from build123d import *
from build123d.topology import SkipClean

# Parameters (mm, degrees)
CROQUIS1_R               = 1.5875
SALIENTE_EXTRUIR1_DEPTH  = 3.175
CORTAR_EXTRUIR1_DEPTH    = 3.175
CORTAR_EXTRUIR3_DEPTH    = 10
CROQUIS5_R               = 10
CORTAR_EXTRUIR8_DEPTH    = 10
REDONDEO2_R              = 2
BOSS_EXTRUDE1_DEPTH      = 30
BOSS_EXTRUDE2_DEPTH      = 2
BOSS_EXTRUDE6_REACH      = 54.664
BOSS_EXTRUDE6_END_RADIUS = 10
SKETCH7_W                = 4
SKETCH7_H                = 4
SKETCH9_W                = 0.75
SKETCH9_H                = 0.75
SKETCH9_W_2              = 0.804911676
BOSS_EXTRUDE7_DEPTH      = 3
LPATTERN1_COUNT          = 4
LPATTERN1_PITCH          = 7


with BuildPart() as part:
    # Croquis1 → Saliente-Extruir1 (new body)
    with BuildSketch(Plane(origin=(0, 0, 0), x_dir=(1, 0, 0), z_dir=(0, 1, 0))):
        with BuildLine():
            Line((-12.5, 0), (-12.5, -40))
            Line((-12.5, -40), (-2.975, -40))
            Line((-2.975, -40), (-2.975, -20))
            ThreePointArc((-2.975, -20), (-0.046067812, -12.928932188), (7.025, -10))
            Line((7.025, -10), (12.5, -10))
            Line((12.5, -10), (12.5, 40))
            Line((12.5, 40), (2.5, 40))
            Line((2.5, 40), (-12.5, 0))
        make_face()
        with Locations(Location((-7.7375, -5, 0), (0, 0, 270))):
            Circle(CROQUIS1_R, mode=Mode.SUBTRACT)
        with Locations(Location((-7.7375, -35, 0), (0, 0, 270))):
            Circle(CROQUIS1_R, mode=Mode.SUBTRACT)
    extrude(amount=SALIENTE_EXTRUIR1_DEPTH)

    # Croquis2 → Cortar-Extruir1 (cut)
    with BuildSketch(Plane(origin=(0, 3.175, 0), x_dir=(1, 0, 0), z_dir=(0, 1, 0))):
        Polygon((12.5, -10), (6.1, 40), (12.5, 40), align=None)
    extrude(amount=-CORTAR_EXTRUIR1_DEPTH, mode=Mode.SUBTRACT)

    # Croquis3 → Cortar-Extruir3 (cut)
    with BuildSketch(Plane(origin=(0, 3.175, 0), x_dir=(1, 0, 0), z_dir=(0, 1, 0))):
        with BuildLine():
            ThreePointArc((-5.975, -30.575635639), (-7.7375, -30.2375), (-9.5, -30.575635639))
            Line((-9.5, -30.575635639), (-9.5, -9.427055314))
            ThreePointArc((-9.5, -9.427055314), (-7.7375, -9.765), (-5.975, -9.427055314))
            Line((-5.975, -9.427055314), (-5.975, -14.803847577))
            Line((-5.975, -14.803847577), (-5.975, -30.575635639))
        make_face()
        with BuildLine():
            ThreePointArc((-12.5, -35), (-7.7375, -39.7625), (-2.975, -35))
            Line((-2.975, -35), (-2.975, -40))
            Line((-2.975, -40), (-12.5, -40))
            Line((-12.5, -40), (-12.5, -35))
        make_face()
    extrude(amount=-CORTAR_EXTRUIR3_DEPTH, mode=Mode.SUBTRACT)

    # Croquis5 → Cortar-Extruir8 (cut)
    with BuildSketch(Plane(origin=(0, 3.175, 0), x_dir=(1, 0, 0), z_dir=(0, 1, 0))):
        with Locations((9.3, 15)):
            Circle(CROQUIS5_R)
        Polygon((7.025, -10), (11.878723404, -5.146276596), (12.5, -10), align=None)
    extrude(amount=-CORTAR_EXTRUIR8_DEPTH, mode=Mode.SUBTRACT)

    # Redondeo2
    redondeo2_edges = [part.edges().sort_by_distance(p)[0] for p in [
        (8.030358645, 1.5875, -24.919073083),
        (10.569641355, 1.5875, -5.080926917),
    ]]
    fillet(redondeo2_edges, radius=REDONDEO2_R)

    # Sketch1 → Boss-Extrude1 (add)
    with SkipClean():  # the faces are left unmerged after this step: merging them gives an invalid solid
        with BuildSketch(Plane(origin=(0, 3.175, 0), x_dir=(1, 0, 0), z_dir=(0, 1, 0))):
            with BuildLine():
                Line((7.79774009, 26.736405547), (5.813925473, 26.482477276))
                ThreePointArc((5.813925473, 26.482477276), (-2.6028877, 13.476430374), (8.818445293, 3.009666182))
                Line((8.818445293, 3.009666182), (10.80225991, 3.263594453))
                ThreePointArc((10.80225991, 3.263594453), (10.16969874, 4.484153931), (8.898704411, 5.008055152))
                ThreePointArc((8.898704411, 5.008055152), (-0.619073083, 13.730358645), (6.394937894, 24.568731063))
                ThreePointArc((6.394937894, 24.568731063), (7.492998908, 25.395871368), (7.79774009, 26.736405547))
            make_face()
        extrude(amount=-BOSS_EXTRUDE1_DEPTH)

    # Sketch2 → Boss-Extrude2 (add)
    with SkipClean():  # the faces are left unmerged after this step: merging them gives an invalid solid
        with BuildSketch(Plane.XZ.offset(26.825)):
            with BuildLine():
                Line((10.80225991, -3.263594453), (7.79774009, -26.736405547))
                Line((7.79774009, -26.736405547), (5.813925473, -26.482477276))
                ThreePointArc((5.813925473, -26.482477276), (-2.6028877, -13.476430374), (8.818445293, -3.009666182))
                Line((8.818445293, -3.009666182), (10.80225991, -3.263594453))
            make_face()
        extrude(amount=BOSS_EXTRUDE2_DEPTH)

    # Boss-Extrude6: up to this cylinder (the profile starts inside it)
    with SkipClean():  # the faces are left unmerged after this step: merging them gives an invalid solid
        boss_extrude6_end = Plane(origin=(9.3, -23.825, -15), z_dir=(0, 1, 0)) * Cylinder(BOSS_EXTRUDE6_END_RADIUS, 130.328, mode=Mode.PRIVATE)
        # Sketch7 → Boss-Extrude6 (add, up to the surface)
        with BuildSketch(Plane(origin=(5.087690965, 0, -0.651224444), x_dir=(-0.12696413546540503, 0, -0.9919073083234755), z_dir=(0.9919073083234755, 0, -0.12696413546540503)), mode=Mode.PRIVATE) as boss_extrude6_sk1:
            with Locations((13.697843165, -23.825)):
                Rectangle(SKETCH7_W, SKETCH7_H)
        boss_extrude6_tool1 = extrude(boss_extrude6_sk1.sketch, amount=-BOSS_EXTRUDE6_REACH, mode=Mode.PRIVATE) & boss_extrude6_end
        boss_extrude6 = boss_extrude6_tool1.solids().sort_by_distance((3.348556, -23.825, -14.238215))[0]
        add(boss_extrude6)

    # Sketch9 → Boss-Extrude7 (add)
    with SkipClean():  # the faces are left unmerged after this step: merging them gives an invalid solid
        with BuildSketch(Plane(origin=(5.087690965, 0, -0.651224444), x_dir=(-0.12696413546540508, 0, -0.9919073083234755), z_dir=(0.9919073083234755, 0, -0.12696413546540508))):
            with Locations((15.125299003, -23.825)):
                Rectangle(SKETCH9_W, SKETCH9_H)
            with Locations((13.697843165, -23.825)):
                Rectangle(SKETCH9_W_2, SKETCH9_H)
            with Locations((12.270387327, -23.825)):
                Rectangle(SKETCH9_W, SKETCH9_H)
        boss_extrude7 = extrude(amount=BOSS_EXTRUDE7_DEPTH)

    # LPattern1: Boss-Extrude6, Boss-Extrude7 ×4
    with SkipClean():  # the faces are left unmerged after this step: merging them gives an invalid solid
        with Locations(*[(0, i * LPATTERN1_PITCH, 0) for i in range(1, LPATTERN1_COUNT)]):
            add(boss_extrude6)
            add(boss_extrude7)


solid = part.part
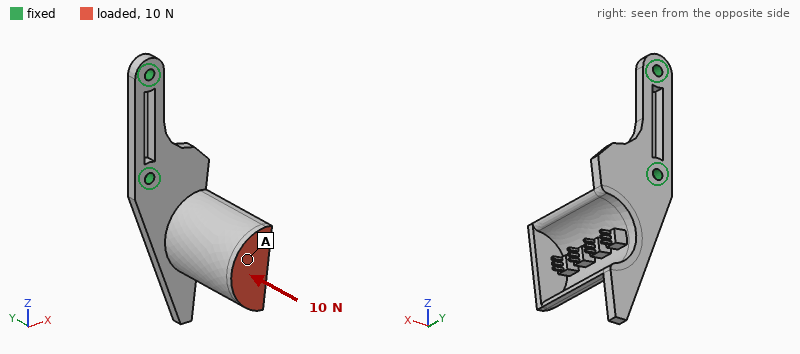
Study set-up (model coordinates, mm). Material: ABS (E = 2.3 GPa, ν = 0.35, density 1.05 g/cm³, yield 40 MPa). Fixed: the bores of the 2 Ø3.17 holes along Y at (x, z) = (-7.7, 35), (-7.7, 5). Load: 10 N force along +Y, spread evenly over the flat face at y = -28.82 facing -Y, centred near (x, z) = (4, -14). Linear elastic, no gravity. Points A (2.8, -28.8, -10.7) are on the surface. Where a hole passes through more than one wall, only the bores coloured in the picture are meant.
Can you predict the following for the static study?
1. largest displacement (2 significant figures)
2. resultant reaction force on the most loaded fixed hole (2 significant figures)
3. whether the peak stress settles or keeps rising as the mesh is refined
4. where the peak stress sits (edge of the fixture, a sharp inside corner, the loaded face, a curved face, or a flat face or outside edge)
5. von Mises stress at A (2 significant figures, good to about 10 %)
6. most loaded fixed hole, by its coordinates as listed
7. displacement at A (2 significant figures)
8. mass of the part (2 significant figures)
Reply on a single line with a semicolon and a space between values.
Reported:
0.99 mm; 11 N; keeps rising; edge of the fixture; 0.82 MPa; (-7.7, 5); 0.76 mm; 5.4 g
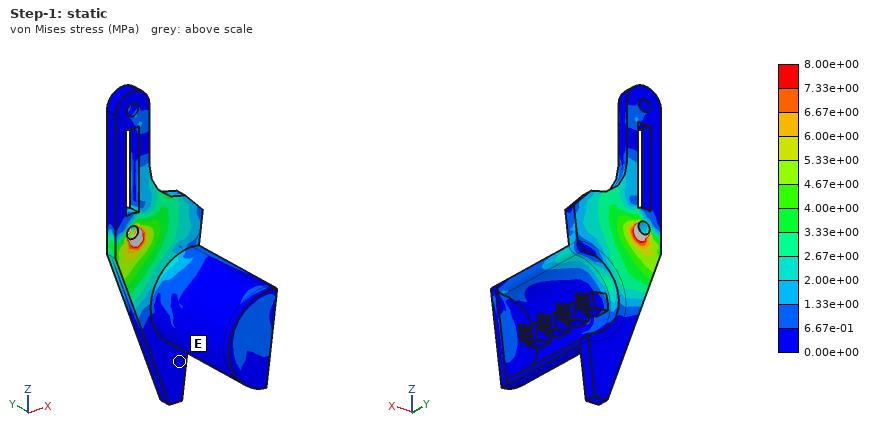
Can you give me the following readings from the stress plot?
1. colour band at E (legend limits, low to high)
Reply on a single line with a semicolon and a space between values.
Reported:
0.00e+00 to 6.67e-01 MPa
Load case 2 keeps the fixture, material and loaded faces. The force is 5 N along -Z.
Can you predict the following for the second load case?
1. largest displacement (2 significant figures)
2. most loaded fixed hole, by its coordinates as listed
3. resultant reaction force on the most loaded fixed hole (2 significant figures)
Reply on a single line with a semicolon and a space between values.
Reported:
0.96 mm; (-7.7, 5); 3.8 N
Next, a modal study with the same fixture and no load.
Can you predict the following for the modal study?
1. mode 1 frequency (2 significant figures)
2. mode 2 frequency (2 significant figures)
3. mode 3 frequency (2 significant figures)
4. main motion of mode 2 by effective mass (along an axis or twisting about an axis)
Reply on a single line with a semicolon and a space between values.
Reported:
270 Hz; 430 Hz; 970 Hz; along X
